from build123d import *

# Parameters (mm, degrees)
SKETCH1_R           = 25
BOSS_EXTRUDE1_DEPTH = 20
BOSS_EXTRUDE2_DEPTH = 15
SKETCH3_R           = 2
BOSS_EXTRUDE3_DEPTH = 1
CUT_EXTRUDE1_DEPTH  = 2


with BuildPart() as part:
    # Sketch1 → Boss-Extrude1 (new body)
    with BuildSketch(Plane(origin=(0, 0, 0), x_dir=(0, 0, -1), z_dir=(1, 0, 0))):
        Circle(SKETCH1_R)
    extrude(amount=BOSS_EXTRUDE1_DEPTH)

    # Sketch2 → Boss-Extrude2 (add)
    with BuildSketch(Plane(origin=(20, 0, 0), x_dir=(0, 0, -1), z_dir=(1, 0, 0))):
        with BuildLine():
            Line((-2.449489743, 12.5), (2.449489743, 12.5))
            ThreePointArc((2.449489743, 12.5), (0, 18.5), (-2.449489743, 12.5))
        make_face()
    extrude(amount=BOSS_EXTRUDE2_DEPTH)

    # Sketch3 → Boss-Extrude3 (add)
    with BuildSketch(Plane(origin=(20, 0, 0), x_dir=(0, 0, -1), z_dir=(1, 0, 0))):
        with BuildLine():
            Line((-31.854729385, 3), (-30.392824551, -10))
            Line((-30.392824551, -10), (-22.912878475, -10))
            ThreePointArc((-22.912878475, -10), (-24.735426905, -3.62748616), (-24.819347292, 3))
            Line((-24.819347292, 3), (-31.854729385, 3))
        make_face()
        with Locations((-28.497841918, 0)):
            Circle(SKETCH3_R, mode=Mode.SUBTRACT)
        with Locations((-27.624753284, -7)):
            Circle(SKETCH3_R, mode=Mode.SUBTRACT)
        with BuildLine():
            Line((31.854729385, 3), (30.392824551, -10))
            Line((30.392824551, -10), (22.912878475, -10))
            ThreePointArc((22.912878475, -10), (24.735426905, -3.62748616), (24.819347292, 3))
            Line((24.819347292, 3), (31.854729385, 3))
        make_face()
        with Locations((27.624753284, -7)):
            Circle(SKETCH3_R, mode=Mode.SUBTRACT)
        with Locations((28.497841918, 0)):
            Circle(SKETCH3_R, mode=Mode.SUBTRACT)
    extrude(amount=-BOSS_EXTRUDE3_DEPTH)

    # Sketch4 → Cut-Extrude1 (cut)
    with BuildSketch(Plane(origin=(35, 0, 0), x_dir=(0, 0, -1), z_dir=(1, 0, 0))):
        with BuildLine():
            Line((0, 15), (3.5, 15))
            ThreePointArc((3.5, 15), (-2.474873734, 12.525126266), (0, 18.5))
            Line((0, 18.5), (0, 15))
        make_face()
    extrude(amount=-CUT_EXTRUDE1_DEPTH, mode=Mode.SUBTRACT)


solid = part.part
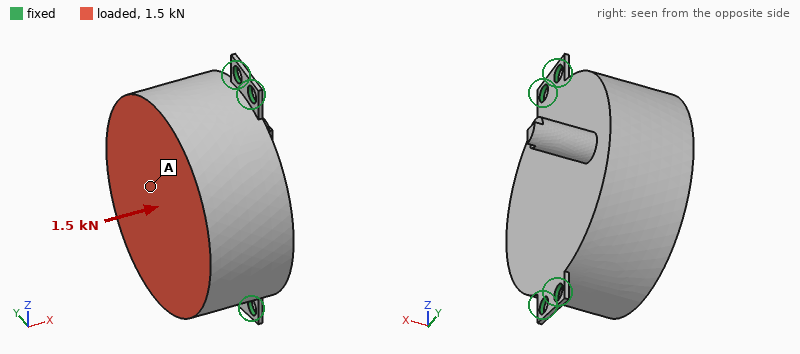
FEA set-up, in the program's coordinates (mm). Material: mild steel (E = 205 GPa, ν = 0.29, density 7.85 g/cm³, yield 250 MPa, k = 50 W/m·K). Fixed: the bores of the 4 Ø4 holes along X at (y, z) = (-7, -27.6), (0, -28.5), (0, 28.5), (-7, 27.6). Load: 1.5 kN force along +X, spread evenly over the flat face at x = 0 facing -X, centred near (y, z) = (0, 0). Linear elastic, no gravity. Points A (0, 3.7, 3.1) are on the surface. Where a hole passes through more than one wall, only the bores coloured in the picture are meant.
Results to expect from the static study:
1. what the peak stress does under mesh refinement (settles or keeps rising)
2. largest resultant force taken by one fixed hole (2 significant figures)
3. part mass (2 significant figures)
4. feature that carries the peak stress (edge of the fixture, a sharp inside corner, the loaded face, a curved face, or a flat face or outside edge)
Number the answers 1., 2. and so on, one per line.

1. keeps rising
2. 790 N
3. 310 g
4. edge of the fixture
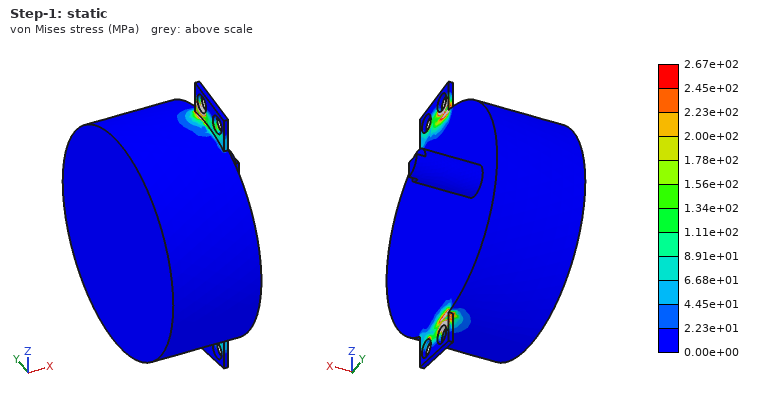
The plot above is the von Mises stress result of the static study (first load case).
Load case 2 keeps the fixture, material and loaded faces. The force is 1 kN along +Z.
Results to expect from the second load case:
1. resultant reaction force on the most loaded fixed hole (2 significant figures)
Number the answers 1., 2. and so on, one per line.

1. 320 N
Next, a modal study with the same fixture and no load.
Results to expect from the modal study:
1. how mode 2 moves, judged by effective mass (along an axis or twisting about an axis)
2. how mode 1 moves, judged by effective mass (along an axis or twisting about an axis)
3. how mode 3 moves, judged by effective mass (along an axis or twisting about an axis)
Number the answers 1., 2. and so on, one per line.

1. along X
2. along Y
3. along Z
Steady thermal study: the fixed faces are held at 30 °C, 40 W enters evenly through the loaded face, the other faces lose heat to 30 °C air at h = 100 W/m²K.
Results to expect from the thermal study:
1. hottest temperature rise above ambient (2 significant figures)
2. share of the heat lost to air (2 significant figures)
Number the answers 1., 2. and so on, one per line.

1. 52 K
2. 62 %
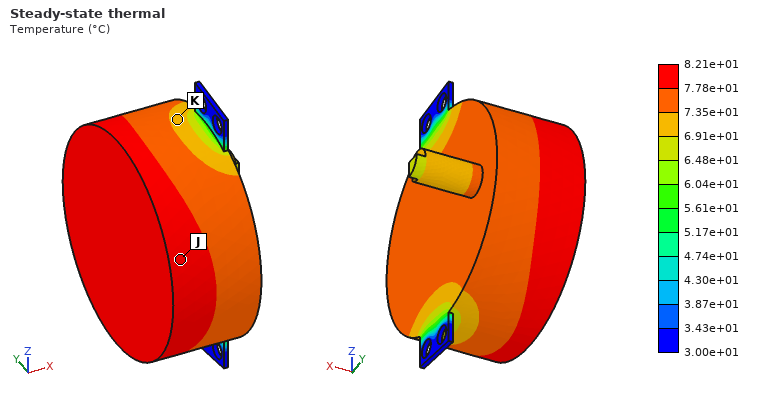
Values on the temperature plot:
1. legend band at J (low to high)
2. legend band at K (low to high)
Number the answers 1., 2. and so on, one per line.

1. 7.78e+01 to 8.21e+01 °C
2. 6.91e+01 to 7.35e+01 °C
